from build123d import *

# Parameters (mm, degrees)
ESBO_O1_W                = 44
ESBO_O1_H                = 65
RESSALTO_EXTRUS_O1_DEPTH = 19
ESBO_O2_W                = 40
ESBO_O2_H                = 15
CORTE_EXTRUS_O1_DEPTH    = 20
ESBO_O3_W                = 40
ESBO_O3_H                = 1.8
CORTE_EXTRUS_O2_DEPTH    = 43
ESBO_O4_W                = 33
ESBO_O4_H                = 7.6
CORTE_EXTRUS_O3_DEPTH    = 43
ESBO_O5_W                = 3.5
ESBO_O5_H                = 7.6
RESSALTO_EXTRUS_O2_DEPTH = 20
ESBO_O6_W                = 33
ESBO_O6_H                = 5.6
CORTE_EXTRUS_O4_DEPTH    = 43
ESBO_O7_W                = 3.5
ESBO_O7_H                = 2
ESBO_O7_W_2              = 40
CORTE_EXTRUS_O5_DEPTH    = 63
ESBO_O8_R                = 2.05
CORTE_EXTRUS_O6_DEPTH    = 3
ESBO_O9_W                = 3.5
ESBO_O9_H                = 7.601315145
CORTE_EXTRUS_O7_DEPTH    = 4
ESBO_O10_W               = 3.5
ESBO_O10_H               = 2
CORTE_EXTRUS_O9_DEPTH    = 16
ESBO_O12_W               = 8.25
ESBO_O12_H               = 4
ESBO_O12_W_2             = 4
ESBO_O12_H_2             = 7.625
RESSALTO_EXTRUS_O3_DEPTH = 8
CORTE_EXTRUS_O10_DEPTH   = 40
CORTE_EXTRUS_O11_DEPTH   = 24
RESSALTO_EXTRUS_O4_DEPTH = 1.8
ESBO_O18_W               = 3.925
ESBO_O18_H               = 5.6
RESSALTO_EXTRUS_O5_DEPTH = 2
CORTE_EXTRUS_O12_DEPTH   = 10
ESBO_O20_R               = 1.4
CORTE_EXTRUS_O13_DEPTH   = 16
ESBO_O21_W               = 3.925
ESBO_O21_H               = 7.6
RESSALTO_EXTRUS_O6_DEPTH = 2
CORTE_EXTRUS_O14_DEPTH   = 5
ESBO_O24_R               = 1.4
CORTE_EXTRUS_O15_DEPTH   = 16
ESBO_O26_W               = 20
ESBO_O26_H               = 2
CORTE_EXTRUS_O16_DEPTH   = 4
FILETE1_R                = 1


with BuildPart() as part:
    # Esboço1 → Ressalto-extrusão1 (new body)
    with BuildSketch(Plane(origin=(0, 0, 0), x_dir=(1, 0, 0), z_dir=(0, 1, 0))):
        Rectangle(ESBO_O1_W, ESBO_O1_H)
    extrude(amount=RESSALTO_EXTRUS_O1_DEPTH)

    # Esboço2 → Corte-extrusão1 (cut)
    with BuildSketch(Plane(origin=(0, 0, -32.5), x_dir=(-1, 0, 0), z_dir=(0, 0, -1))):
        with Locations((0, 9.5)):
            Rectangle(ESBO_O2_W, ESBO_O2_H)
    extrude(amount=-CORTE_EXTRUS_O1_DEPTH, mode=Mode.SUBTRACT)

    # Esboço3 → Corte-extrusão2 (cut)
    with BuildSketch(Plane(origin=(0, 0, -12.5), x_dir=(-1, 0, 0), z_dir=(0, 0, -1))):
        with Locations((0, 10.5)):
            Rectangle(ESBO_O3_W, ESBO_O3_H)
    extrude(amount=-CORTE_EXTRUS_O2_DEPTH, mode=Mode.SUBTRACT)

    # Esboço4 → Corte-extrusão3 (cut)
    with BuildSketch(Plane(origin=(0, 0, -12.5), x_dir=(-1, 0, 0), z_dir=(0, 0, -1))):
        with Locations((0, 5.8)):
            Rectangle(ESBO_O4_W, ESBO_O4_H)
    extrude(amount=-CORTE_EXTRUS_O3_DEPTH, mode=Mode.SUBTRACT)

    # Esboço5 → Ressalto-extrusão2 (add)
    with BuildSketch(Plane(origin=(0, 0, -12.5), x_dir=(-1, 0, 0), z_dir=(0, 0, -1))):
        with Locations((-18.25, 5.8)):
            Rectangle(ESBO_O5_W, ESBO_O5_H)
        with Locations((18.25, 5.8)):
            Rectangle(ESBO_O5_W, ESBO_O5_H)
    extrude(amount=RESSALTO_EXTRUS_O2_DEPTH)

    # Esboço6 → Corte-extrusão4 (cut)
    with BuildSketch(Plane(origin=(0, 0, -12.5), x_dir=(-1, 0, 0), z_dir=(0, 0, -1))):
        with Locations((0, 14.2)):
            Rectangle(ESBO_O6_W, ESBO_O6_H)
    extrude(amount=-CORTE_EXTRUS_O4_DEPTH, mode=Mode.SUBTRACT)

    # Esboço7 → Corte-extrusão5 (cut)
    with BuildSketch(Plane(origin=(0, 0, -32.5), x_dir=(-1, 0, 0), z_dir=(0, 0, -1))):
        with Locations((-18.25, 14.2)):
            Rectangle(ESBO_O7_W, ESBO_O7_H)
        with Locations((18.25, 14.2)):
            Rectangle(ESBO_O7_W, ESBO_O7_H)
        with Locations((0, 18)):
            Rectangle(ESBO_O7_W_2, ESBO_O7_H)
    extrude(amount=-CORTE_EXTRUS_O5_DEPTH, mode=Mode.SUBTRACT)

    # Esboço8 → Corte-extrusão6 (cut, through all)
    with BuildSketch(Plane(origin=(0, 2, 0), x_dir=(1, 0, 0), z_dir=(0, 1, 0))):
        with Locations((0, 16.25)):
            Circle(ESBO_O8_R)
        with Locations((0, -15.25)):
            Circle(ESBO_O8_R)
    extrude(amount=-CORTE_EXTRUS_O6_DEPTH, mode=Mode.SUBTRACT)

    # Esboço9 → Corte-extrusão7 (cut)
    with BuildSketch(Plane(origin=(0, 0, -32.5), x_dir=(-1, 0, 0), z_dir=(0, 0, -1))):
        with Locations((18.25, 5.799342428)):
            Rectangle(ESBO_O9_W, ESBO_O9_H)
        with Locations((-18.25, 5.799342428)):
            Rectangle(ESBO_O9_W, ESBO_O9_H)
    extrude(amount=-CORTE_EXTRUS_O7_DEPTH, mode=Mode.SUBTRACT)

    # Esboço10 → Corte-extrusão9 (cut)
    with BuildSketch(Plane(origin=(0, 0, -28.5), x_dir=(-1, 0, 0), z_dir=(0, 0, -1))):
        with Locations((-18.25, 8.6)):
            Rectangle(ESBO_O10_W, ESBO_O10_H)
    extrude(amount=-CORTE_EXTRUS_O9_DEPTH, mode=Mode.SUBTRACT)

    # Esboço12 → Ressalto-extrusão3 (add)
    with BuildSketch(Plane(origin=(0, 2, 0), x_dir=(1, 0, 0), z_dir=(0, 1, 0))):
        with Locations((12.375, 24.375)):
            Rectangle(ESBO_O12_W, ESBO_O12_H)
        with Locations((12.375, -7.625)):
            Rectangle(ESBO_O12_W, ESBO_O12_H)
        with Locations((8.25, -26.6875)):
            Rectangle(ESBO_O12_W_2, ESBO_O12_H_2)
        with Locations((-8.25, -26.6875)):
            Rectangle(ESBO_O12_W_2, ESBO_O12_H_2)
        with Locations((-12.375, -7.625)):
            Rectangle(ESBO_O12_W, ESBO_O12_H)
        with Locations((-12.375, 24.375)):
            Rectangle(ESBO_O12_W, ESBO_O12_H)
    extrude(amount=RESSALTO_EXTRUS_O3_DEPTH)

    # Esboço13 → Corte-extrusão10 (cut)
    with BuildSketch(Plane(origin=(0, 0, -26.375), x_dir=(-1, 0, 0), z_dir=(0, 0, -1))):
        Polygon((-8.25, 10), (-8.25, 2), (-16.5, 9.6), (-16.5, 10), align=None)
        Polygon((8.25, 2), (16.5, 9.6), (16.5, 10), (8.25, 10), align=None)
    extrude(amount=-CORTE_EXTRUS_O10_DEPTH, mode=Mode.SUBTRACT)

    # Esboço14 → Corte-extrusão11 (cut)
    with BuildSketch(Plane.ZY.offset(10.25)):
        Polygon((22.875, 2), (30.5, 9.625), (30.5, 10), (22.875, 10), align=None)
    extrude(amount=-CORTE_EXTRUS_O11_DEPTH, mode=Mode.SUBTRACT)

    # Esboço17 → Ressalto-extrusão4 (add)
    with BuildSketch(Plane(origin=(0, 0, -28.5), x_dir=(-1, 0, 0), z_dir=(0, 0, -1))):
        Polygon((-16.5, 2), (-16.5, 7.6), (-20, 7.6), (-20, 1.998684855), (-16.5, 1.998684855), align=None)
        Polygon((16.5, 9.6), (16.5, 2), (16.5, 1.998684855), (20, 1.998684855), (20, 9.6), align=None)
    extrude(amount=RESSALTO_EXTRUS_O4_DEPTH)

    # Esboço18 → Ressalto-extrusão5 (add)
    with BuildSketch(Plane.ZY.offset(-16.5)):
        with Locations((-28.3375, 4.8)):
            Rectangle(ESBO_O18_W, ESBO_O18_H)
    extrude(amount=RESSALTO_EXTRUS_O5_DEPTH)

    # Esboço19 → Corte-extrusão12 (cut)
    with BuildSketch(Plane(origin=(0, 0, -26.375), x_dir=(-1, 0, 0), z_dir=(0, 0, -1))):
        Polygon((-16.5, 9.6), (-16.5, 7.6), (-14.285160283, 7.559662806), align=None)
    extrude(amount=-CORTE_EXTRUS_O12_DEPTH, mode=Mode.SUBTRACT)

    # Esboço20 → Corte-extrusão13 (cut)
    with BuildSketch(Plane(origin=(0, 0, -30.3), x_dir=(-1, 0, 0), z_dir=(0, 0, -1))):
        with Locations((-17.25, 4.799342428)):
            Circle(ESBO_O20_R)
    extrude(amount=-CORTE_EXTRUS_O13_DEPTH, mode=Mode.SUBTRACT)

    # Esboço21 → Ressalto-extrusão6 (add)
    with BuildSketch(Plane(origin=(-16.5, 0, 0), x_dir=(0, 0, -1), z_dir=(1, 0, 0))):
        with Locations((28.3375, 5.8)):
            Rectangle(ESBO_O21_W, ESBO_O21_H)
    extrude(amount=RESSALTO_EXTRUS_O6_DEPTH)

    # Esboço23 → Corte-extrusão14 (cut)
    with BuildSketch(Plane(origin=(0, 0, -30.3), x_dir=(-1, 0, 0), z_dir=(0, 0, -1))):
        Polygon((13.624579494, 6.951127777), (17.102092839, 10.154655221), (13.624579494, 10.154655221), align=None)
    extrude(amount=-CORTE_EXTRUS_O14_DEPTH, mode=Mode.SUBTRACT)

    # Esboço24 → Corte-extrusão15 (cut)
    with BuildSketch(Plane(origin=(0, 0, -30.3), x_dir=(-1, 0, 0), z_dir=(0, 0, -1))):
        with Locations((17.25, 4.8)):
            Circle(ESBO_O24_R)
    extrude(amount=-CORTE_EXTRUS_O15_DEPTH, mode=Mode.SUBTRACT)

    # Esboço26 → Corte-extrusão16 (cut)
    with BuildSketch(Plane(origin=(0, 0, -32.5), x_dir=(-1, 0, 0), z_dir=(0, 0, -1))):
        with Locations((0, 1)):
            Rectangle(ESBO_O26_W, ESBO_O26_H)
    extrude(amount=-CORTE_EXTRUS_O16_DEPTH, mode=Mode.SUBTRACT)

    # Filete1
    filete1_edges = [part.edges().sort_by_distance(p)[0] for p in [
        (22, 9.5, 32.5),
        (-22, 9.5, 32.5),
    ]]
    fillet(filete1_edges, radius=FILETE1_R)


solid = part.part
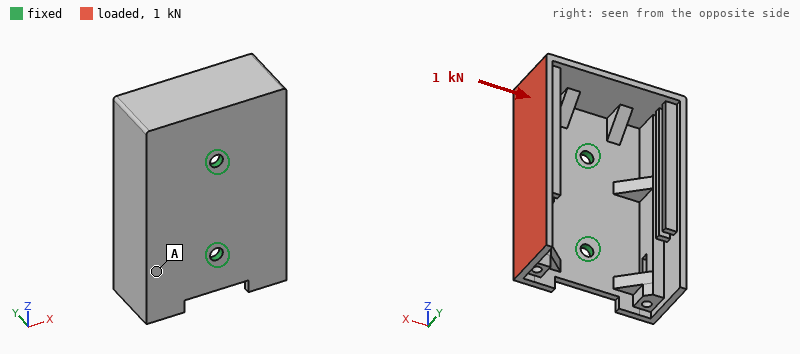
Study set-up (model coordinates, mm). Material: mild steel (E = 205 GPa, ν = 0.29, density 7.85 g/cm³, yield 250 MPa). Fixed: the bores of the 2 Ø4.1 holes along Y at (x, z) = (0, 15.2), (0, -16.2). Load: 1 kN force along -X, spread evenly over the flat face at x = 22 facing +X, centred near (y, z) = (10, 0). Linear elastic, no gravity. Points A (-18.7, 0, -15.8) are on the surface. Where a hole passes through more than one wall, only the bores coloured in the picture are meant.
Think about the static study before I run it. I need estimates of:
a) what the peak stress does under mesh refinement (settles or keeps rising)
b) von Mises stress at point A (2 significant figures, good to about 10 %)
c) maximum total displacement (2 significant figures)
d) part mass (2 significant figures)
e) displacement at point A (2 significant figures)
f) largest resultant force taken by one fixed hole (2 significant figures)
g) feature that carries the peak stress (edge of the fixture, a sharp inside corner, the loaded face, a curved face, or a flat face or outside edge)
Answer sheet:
keeps rising
22 MPa
0.20 mm
130 g
0.048 mm
510 N
edge of the fixture
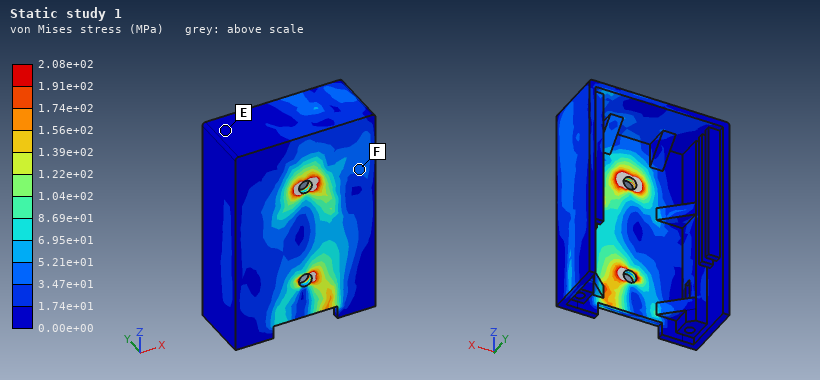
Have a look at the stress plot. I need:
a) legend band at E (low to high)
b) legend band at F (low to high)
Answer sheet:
0.00e+00 to 1.74e+01 MPa
3.47e+01 to 5.21e+01 MPa
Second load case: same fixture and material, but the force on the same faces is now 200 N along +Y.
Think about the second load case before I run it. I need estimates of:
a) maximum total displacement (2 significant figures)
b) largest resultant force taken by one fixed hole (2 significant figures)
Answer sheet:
81 µm
100 N
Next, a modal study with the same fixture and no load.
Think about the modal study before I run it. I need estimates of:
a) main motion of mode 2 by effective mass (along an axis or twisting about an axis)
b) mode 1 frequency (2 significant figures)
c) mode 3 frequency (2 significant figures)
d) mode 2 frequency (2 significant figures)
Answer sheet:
along Y
1100 Hz
2800 Hz
2100 Hz
